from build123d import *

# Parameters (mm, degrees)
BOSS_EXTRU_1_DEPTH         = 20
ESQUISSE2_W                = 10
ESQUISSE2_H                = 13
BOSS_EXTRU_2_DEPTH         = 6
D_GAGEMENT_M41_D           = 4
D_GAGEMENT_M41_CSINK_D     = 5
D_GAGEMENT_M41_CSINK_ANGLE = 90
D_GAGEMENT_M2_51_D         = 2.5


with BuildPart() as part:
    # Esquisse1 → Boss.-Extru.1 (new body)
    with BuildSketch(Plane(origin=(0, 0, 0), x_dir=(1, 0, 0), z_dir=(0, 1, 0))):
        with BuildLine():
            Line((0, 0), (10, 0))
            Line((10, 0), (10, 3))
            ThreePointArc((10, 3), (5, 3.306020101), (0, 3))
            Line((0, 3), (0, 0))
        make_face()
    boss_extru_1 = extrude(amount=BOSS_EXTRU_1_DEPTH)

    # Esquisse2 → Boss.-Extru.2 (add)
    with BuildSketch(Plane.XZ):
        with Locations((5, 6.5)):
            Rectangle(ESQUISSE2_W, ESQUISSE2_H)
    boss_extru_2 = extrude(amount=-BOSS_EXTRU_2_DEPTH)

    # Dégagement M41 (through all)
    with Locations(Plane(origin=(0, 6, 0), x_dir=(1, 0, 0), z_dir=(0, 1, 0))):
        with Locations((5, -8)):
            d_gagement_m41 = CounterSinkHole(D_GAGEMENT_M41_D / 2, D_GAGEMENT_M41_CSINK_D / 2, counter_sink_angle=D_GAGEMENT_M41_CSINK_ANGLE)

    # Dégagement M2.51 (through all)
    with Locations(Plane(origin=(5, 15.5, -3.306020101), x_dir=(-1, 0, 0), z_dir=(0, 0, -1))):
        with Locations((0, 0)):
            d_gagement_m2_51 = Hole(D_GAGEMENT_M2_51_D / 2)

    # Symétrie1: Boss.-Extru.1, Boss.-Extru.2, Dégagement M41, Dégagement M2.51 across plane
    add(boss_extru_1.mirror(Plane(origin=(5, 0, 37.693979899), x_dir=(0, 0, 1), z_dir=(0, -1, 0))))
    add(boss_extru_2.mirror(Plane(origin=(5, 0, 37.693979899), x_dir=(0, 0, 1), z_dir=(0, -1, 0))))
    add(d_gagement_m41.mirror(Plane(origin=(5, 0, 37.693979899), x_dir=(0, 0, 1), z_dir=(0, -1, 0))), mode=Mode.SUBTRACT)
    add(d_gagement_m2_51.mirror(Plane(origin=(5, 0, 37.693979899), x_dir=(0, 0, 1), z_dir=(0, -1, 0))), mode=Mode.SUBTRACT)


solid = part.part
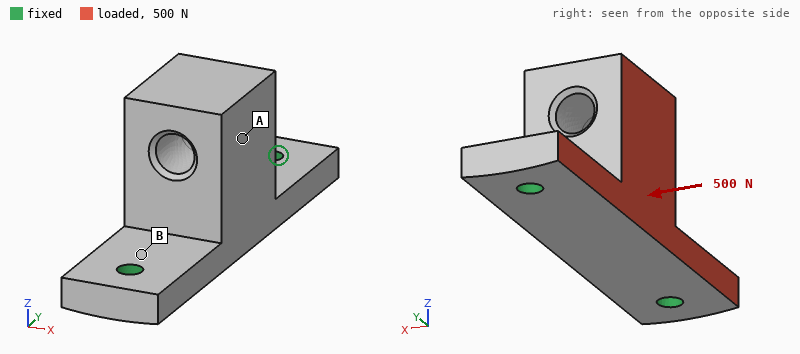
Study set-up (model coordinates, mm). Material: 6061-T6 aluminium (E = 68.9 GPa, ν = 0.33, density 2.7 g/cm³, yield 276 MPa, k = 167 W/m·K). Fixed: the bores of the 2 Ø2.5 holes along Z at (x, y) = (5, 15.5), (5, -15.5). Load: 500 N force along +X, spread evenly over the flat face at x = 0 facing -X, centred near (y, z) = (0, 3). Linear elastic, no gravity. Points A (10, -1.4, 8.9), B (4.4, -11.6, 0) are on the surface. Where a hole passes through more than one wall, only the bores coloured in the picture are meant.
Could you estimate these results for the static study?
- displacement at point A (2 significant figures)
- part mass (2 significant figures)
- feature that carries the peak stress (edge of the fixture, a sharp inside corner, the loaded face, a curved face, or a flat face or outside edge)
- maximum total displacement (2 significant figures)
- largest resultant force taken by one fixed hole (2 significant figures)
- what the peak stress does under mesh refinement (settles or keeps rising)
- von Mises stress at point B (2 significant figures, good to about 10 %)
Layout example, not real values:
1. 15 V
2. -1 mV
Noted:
1. 61 µm
2. 7.2 g
3. edge of the fixture
4. 79 µm
5. 250 N
6. keeps rising
7. 75 MPa
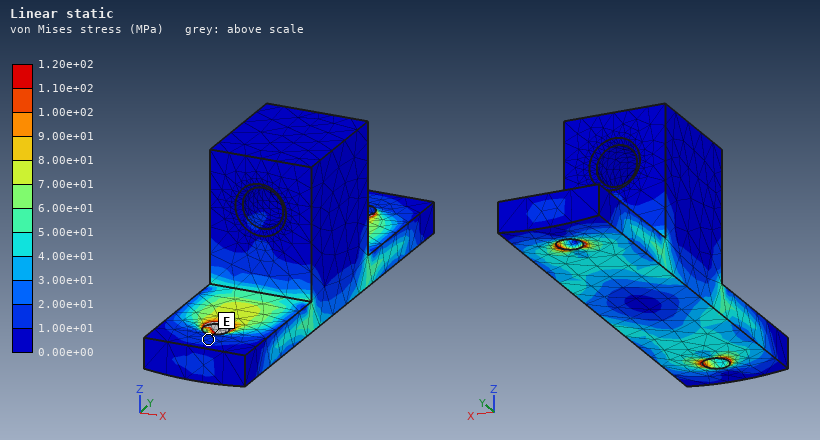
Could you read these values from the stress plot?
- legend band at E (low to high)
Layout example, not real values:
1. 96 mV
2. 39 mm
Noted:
1. 1.00e+01 to 2.00e+01 MPa
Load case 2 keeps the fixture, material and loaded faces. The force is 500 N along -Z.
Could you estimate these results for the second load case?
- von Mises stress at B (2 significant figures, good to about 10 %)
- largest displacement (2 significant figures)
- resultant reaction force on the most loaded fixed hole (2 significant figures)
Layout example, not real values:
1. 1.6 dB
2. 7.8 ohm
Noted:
1. 55 MPa
2. 67 µm
3. 260 N
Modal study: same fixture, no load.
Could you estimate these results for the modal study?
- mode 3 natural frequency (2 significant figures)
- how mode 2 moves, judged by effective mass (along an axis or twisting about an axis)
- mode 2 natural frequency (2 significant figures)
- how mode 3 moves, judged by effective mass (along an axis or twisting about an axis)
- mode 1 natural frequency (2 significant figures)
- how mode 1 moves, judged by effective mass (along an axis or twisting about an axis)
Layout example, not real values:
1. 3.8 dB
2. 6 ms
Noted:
1. 14 kHz
2. along Z
3. 11 kHz
4. along Y
5. 5800 Hz
6. along X
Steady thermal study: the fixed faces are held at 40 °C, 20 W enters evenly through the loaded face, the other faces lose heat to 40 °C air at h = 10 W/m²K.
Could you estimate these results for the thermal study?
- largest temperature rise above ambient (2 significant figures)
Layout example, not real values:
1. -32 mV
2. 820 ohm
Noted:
1. 23 K
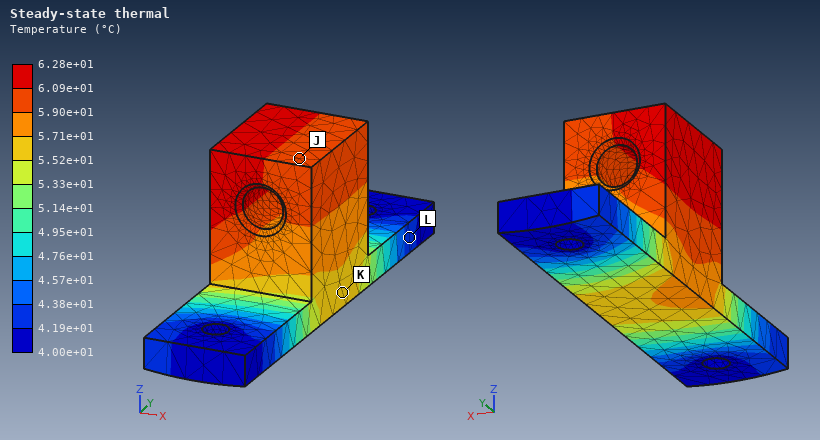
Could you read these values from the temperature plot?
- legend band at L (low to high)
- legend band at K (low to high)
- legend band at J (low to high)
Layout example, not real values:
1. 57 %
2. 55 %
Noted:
1. 4.19e+01 to 4.38e+01 °C
2. 5.52e+01 to 5.71e+01 °C
3. 5.90e+01 to 6.09e+01 °C
